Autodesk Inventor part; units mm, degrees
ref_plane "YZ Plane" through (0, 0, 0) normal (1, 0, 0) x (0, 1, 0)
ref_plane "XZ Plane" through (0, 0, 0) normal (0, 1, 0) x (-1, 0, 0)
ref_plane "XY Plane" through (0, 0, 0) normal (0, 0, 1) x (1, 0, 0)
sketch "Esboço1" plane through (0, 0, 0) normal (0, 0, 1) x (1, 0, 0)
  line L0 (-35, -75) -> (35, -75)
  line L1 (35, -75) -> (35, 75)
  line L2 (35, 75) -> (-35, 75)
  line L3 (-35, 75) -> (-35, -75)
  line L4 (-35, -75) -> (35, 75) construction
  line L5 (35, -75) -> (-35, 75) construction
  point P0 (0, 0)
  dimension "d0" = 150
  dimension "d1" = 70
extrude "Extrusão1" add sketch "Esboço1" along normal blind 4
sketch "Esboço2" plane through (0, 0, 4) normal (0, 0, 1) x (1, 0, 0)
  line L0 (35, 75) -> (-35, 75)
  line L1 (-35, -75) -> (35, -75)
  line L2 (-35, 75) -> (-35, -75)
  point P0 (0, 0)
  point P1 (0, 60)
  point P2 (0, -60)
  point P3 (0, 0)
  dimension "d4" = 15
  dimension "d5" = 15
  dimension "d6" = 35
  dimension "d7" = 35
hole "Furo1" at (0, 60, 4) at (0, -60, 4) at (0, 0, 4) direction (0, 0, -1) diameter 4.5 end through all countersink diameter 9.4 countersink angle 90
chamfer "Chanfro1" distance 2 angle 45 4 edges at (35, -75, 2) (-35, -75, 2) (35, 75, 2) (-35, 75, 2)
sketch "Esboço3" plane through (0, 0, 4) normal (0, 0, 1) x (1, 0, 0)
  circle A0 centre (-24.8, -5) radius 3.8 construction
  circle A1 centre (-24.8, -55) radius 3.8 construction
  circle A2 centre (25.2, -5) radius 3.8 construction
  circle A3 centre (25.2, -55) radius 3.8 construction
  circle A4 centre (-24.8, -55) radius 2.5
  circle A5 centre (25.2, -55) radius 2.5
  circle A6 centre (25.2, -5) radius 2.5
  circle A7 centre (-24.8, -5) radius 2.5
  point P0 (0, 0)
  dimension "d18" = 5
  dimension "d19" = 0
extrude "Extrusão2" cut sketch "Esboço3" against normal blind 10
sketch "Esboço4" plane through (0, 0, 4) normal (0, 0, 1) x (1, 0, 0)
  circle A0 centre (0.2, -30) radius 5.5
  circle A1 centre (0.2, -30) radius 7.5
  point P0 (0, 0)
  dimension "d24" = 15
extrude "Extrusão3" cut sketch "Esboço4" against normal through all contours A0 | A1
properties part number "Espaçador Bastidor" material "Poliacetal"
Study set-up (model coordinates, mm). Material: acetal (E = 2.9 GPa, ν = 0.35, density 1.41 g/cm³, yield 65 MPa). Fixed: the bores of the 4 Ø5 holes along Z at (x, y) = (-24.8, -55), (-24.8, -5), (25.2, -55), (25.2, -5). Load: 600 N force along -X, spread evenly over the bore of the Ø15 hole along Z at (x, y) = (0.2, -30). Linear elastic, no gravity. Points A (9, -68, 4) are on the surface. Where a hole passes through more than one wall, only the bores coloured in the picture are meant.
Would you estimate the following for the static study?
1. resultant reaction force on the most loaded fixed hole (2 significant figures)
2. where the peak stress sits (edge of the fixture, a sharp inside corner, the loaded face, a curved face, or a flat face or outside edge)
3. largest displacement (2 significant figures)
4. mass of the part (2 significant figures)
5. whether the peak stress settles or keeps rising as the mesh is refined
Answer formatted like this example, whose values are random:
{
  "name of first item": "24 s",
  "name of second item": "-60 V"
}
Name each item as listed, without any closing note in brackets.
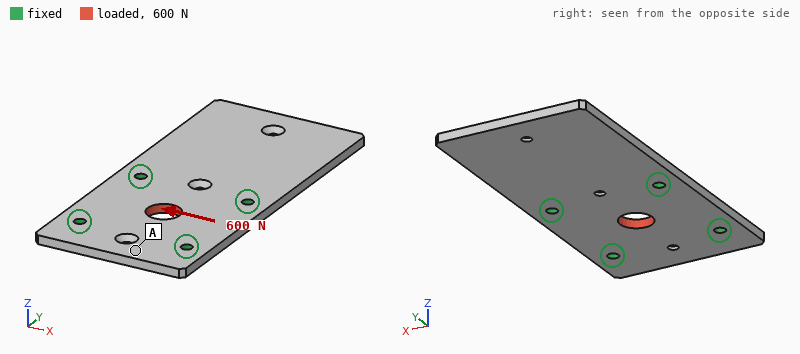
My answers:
{
  "resultant reaction force on the most loaded fixed hole": "170 N",
  "where the peak stress sits": "edge of the fixture",
  "largest displacement": "34 µm",
  "mass of the part": "57 g",
  "whether the peak stress settles or keeps rising as the mesh is refined": "keeps rising"
}
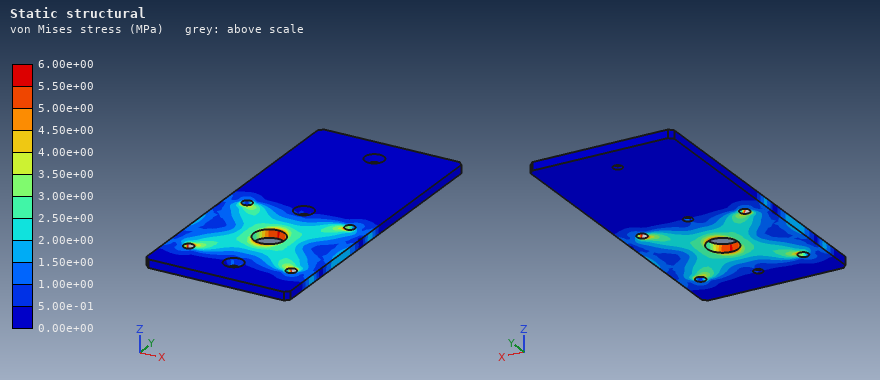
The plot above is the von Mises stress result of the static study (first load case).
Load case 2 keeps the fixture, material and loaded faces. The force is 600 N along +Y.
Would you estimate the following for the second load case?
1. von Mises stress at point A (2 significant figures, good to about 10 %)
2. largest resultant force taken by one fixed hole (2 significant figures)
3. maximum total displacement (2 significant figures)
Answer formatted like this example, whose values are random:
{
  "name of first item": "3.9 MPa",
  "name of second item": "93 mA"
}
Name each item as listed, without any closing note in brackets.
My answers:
{
  "von Mises stress at point A": "0.89 MPa",
  "largest resultant force taken by one fixed hole": "160 N",
  "maximum total displacement": "30 µm"
}
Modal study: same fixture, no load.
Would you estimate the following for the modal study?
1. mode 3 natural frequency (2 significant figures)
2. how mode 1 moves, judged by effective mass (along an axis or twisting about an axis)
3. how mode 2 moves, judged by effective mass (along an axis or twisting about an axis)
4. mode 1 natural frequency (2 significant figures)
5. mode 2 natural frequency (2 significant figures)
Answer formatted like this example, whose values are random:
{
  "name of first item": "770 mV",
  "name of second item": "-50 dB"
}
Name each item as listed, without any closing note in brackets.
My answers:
{
  "mode 3 natural frequency": "880 Hz",
  "how mode 1 moves, judged by effective mass": "along Z",
  "how mode 2 moves, judged by effective mass": "twisting about Y",
  "mode 1 natural frequency": "140 Hz",
  "mode 2 natural frequency": "390 Hz"
}
